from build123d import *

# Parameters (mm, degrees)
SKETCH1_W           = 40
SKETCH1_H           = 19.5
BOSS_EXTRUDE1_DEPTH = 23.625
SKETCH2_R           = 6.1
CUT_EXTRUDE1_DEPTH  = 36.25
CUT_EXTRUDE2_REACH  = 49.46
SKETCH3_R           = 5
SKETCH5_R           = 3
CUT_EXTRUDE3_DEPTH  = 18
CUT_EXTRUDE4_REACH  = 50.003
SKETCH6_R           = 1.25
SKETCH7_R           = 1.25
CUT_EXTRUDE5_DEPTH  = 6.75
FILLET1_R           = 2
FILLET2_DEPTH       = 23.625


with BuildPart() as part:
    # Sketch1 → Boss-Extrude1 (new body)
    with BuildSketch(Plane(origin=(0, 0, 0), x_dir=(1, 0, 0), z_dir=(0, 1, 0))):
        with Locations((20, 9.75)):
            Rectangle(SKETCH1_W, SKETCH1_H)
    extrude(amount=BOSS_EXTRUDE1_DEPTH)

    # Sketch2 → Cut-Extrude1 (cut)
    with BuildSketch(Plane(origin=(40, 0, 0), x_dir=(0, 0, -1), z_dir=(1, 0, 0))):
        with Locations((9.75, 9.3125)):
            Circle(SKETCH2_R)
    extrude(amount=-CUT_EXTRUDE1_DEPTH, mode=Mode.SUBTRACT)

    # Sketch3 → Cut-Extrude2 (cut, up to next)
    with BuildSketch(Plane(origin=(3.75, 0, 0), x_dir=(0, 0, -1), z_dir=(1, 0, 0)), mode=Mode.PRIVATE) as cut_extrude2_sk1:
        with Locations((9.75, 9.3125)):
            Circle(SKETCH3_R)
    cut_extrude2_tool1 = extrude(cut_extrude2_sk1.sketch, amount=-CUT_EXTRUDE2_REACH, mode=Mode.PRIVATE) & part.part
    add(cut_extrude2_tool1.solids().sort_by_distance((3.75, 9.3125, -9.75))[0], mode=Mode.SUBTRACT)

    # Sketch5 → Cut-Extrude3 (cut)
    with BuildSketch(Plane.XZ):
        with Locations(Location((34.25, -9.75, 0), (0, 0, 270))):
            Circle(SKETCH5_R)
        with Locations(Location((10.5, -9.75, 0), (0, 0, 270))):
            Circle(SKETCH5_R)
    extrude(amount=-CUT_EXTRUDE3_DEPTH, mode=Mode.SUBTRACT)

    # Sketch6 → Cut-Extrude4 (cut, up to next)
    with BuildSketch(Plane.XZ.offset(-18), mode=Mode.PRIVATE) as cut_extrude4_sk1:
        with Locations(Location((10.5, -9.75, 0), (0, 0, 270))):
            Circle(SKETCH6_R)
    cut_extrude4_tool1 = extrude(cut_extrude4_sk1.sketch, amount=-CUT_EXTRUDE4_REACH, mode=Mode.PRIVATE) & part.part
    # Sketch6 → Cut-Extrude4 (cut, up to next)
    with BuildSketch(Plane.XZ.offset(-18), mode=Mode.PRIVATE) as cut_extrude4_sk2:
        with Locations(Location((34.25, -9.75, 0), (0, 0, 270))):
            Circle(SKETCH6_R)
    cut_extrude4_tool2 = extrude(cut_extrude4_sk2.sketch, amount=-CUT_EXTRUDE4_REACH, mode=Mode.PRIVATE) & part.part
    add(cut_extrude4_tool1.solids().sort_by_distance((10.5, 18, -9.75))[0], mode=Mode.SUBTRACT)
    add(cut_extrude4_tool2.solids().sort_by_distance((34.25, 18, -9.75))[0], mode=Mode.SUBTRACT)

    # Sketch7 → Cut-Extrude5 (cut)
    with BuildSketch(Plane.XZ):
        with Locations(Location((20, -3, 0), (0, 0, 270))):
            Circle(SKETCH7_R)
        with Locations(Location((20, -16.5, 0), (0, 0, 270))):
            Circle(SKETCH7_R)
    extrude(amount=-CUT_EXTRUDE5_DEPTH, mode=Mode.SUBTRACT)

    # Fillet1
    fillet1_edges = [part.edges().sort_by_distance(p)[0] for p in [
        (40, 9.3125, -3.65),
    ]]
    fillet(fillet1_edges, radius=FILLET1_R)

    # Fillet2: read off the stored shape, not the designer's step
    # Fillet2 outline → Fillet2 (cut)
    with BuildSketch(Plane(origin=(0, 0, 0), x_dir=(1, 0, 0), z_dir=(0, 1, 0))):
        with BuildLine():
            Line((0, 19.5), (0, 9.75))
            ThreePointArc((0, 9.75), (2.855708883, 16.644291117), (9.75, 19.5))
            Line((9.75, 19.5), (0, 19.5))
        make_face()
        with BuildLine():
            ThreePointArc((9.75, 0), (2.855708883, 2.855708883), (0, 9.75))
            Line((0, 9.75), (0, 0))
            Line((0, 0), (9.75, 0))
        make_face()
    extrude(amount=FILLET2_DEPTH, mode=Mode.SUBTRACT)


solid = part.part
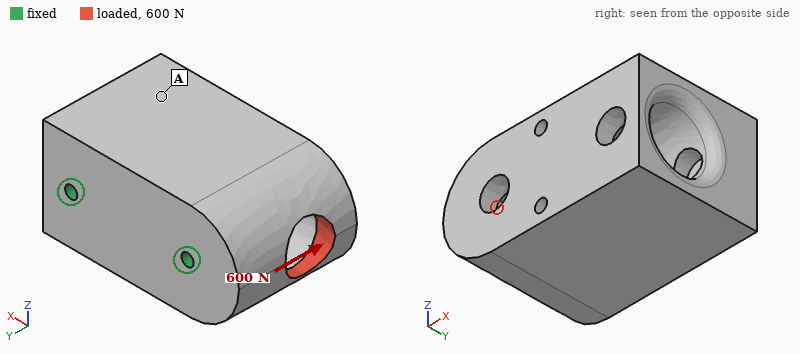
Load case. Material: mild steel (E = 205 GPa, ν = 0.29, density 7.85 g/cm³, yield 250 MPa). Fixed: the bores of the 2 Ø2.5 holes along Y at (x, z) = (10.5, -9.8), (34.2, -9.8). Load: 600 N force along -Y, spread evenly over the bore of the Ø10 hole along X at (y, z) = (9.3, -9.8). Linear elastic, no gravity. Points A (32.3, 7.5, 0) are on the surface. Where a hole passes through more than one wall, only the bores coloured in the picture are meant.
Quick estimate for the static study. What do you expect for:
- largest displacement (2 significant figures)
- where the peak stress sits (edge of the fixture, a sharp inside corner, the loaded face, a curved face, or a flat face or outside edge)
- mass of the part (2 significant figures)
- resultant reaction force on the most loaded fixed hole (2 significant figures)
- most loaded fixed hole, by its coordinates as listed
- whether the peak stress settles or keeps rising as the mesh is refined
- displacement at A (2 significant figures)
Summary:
3.0 µm
edge of the fixture
98 g
760 N
(10.5, -9.8)
keeps rising
0.54 µm
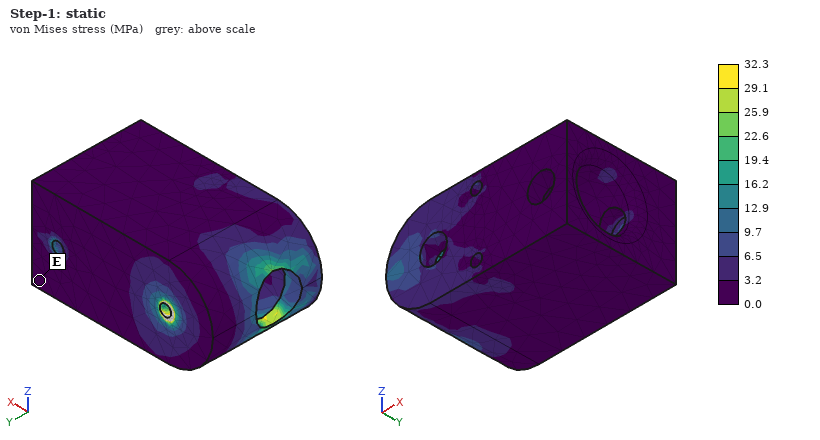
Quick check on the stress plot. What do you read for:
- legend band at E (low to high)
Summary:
0.0 to 3.2 MPa
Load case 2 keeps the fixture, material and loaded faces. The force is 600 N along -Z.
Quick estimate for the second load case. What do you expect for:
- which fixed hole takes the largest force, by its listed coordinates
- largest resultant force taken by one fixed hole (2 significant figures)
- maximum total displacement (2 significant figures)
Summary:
(10.5, -9.8)
780 N
7.8 µm
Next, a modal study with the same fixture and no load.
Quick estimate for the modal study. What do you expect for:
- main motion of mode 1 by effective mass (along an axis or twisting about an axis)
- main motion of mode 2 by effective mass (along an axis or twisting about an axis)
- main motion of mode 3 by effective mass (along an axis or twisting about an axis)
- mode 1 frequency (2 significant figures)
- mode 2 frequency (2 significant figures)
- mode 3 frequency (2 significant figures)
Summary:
along Z
along X
twisting about Y
6400 Hz
16 kHz
21 kHz
